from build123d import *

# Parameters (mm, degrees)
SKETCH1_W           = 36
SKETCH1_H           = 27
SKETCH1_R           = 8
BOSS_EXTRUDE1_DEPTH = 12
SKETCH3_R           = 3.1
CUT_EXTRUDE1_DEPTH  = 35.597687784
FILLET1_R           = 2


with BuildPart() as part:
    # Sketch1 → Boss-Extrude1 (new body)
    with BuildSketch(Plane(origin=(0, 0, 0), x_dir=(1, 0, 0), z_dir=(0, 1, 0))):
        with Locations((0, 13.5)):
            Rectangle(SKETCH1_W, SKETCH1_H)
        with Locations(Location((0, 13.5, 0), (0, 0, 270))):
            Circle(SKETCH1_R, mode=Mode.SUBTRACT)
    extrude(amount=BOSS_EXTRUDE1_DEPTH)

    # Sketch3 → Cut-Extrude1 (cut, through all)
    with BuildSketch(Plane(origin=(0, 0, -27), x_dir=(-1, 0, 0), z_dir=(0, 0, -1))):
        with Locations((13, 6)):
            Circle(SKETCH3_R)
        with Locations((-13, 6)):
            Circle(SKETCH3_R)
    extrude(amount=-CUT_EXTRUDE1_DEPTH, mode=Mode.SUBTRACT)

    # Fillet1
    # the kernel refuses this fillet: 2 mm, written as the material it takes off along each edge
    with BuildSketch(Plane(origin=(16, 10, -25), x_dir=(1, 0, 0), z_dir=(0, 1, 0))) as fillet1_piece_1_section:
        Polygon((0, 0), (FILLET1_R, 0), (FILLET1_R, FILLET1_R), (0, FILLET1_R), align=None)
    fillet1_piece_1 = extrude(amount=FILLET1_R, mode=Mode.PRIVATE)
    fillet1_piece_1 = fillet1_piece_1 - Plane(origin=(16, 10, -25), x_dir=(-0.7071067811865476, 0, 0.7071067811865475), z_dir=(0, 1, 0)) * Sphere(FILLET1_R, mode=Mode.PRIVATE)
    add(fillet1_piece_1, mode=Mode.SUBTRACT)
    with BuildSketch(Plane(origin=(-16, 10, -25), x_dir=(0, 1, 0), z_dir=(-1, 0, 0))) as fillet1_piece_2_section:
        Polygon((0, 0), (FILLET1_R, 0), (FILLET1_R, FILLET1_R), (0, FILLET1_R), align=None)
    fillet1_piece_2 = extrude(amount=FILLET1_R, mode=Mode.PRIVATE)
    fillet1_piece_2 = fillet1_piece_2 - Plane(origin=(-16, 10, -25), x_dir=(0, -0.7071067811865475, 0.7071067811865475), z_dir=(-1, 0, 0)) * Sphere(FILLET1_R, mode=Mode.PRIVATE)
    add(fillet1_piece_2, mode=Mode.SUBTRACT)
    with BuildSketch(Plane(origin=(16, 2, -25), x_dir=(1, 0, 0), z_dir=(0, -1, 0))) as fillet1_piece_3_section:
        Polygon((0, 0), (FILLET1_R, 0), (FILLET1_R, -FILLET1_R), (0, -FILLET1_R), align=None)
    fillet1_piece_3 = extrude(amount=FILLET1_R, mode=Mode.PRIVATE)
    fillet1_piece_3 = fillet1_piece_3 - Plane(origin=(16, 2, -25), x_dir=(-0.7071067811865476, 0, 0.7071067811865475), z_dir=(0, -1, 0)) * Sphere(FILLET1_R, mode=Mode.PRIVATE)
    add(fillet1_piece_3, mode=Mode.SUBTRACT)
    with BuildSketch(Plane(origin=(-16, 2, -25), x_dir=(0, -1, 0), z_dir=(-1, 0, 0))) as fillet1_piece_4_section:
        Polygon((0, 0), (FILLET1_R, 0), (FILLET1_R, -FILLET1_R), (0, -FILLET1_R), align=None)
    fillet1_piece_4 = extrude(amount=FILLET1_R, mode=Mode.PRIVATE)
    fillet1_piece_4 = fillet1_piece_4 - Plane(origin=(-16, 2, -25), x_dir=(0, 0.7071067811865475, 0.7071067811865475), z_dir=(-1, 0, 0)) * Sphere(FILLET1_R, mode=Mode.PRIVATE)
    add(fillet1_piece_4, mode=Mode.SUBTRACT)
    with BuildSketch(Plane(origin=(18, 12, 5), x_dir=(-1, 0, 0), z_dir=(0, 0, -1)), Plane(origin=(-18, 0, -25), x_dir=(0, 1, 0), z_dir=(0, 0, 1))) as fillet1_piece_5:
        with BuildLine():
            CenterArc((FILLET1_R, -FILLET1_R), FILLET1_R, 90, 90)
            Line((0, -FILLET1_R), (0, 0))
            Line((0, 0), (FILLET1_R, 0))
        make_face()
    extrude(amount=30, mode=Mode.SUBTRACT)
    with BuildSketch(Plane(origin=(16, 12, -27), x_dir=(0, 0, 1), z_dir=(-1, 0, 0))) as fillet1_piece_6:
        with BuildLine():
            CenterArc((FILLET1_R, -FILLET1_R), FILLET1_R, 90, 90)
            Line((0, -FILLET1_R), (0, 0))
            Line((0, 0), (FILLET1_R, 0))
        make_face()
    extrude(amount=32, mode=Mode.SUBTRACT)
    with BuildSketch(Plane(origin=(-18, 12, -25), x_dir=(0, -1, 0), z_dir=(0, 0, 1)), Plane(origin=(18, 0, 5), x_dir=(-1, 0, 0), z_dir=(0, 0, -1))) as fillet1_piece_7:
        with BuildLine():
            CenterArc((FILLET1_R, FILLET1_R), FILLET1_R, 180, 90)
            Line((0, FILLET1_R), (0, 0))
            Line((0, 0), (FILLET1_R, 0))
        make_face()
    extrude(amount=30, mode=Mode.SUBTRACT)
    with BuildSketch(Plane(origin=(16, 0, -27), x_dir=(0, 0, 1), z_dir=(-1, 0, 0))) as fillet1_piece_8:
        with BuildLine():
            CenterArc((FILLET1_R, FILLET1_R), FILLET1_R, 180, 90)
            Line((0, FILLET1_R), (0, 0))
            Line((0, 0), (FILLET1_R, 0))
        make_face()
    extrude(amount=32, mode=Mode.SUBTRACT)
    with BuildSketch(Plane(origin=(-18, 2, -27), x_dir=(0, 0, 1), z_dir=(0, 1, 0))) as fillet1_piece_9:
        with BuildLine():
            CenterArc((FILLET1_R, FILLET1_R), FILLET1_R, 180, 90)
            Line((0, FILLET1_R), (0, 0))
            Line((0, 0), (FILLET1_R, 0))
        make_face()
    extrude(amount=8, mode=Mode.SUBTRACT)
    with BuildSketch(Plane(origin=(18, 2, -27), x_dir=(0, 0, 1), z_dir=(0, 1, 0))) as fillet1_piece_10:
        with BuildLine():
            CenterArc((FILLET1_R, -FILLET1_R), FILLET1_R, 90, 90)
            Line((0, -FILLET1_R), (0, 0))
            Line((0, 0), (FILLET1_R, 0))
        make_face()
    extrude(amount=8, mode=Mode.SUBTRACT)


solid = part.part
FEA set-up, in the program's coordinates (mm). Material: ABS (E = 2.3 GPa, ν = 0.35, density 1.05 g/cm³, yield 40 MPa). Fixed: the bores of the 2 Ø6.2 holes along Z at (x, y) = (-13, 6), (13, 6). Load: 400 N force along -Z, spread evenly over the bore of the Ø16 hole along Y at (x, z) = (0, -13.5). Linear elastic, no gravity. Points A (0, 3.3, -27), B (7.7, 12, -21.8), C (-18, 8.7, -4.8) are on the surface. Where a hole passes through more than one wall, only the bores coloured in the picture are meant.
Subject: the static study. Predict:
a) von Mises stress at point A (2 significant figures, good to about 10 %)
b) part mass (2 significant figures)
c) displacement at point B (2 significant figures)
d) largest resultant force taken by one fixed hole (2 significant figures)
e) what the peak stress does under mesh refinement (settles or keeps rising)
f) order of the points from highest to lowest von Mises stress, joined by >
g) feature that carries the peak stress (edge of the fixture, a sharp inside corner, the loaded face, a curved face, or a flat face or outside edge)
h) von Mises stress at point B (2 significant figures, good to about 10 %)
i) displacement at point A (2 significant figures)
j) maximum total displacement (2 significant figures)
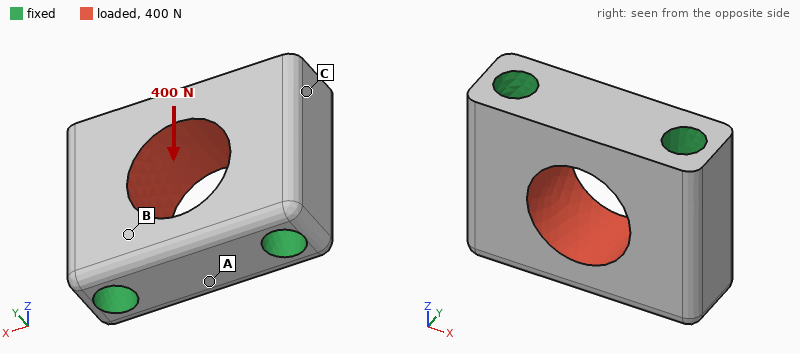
1.4 MPa
7.8 g
2.8 µm
200 N
keeps rising
A > B > C
edge of the fixture
0.86 MPa
8.0 µm
9.8 µm
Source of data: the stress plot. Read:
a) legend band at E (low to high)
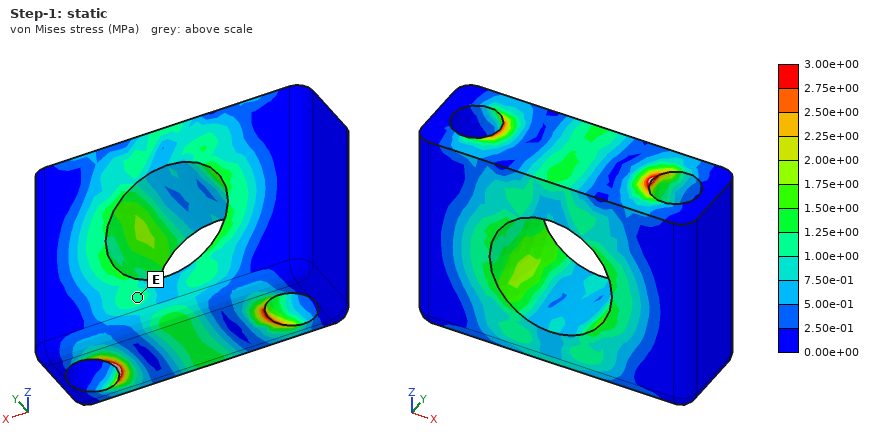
1.00e+00 to 1.25e+00 MPa
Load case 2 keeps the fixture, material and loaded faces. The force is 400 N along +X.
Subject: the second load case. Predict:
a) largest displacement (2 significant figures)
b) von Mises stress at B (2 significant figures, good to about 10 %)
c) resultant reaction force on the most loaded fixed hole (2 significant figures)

3.2 µm
0.55 MPa
200 N
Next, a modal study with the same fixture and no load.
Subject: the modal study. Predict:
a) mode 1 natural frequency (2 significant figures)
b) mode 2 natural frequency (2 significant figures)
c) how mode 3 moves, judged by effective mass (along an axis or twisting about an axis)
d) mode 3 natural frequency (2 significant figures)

17 kHz
18 kHz
along Z
20 kHz
